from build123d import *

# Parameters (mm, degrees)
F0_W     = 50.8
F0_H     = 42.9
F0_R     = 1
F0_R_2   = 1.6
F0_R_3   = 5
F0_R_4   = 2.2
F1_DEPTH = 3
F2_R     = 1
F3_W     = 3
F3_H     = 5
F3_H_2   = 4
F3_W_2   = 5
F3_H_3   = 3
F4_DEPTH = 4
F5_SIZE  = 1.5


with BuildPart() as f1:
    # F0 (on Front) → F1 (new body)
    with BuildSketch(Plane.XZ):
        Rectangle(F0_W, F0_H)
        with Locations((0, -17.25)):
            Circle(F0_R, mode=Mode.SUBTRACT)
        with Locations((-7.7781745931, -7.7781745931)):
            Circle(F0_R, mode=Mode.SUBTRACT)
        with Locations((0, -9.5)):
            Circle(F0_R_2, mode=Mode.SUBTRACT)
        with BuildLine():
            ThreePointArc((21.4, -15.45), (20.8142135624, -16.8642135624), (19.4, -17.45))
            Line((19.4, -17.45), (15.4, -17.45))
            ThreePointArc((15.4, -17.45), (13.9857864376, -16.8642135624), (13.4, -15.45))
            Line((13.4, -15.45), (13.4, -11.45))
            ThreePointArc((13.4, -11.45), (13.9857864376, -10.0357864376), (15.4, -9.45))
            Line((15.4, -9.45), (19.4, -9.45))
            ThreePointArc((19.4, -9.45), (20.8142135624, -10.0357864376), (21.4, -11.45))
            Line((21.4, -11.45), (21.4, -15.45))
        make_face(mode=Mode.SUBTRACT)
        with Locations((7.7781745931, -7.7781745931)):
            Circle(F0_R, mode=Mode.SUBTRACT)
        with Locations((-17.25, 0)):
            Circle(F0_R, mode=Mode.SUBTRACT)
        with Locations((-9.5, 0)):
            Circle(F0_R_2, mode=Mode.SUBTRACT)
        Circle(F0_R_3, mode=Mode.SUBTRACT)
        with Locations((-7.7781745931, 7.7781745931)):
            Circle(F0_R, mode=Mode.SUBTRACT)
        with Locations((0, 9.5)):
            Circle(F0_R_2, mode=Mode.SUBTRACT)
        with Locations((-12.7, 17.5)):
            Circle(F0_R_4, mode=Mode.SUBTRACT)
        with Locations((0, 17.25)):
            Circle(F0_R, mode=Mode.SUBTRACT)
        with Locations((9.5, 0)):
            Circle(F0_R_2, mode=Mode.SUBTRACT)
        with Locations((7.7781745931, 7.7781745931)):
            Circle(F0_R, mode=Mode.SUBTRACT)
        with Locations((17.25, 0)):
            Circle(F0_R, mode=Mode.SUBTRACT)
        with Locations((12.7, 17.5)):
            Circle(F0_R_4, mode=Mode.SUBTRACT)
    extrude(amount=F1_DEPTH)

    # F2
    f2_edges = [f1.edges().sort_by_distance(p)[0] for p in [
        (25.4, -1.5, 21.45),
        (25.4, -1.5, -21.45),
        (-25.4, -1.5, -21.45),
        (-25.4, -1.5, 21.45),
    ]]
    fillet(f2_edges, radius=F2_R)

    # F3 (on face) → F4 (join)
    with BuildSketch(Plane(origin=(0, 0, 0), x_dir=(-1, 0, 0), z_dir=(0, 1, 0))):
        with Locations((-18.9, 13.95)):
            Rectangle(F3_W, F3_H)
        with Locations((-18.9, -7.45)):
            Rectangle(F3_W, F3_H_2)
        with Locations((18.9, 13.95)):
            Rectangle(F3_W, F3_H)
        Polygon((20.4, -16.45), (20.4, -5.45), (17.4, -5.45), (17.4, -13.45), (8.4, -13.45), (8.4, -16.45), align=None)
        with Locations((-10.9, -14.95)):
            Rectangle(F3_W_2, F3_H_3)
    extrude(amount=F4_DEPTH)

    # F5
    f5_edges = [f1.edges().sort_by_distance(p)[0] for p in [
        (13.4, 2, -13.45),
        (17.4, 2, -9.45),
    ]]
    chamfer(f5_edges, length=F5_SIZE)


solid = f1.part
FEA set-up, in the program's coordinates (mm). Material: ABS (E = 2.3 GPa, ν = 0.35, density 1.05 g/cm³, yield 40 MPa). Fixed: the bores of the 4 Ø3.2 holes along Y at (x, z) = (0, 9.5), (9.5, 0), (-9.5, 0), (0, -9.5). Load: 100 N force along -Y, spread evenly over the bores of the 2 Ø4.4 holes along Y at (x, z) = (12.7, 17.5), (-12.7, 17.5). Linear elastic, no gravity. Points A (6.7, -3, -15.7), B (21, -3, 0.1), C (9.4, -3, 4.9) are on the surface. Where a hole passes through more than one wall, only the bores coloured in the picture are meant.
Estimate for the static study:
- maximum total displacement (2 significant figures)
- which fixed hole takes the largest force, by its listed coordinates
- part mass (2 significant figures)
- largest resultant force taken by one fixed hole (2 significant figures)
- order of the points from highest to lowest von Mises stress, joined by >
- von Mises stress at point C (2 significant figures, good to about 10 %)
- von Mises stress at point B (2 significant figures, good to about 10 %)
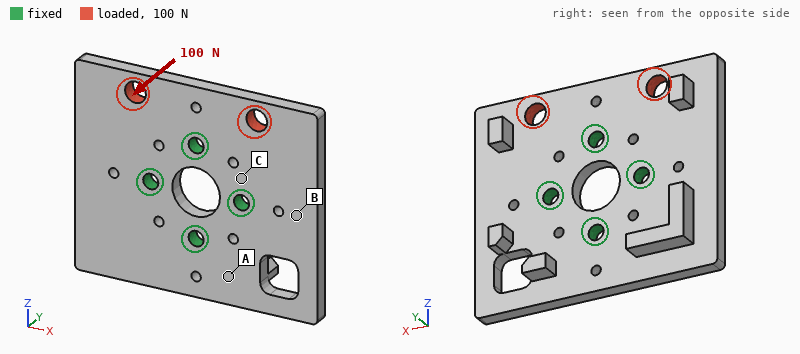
0.61 mm
(0, 9.5)
6.6 g
83 N
C > B > A
9.6 MPa
5.3 MPa
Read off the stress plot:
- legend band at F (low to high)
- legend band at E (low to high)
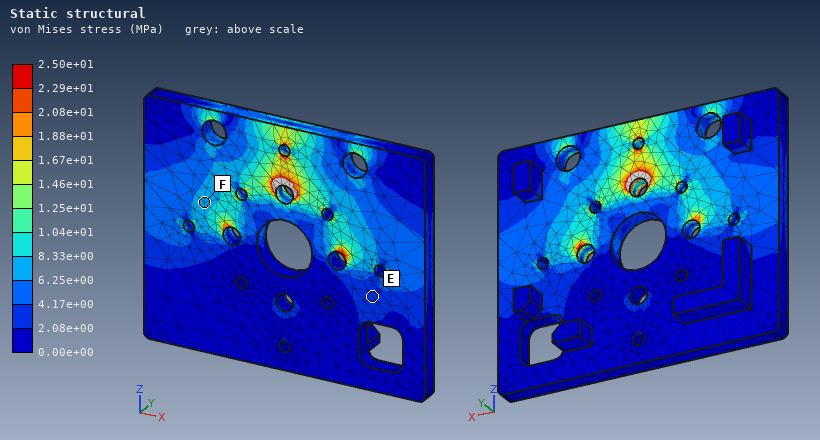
6.25e+00 to 8.33e+00 MPa
2.08e+00 to 4.17e+00 MPa
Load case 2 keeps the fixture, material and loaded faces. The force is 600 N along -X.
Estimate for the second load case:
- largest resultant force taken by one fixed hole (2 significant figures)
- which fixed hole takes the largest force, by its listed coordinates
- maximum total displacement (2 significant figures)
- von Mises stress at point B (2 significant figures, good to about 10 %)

560 N
(0, 9.5)
0.17 mm
2.5 MPa
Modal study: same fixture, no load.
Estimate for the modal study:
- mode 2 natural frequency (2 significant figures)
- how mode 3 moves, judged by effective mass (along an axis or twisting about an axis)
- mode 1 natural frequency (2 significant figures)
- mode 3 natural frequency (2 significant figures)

1700 Hz
along Y
1600 Hz
1800 Hz
